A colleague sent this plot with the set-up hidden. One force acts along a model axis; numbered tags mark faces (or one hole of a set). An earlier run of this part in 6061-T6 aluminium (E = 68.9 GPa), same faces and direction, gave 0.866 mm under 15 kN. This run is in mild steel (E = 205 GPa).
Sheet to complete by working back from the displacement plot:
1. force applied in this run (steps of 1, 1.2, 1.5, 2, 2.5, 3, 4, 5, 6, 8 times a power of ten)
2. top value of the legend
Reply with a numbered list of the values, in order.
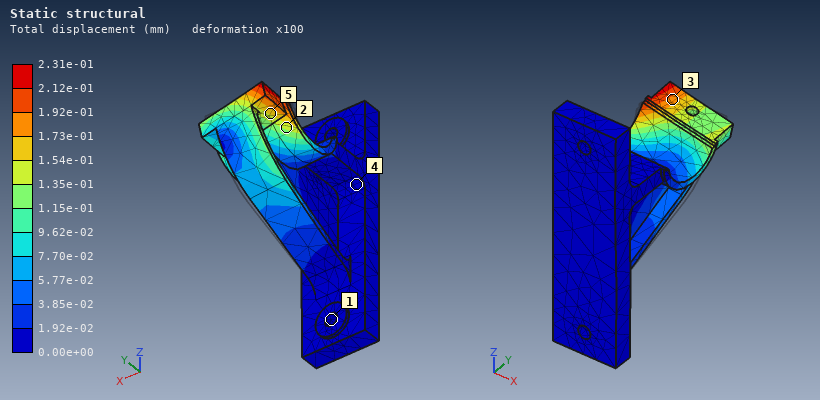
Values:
1. 12 kN
2. 2.31e-01 mm
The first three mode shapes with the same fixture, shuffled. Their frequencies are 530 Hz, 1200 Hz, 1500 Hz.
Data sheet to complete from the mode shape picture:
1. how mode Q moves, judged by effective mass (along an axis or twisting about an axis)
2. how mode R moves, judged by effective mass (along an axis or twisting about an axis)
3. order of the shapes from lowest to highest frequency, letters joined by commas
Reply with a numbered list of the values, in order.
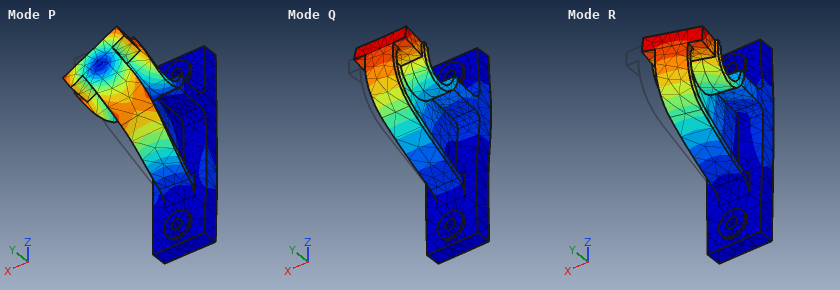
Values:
1. along Z
2. along X
3. R, P, Q
